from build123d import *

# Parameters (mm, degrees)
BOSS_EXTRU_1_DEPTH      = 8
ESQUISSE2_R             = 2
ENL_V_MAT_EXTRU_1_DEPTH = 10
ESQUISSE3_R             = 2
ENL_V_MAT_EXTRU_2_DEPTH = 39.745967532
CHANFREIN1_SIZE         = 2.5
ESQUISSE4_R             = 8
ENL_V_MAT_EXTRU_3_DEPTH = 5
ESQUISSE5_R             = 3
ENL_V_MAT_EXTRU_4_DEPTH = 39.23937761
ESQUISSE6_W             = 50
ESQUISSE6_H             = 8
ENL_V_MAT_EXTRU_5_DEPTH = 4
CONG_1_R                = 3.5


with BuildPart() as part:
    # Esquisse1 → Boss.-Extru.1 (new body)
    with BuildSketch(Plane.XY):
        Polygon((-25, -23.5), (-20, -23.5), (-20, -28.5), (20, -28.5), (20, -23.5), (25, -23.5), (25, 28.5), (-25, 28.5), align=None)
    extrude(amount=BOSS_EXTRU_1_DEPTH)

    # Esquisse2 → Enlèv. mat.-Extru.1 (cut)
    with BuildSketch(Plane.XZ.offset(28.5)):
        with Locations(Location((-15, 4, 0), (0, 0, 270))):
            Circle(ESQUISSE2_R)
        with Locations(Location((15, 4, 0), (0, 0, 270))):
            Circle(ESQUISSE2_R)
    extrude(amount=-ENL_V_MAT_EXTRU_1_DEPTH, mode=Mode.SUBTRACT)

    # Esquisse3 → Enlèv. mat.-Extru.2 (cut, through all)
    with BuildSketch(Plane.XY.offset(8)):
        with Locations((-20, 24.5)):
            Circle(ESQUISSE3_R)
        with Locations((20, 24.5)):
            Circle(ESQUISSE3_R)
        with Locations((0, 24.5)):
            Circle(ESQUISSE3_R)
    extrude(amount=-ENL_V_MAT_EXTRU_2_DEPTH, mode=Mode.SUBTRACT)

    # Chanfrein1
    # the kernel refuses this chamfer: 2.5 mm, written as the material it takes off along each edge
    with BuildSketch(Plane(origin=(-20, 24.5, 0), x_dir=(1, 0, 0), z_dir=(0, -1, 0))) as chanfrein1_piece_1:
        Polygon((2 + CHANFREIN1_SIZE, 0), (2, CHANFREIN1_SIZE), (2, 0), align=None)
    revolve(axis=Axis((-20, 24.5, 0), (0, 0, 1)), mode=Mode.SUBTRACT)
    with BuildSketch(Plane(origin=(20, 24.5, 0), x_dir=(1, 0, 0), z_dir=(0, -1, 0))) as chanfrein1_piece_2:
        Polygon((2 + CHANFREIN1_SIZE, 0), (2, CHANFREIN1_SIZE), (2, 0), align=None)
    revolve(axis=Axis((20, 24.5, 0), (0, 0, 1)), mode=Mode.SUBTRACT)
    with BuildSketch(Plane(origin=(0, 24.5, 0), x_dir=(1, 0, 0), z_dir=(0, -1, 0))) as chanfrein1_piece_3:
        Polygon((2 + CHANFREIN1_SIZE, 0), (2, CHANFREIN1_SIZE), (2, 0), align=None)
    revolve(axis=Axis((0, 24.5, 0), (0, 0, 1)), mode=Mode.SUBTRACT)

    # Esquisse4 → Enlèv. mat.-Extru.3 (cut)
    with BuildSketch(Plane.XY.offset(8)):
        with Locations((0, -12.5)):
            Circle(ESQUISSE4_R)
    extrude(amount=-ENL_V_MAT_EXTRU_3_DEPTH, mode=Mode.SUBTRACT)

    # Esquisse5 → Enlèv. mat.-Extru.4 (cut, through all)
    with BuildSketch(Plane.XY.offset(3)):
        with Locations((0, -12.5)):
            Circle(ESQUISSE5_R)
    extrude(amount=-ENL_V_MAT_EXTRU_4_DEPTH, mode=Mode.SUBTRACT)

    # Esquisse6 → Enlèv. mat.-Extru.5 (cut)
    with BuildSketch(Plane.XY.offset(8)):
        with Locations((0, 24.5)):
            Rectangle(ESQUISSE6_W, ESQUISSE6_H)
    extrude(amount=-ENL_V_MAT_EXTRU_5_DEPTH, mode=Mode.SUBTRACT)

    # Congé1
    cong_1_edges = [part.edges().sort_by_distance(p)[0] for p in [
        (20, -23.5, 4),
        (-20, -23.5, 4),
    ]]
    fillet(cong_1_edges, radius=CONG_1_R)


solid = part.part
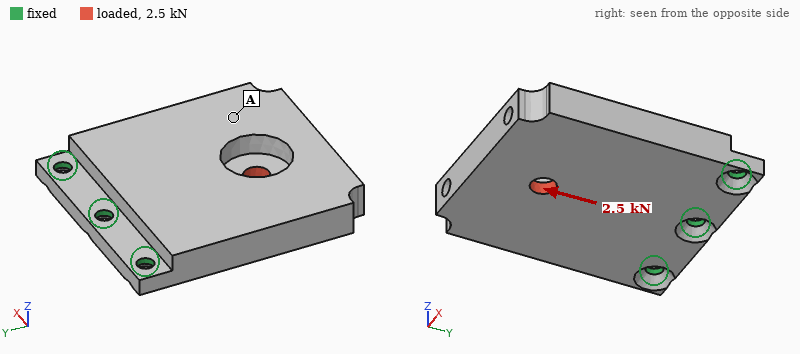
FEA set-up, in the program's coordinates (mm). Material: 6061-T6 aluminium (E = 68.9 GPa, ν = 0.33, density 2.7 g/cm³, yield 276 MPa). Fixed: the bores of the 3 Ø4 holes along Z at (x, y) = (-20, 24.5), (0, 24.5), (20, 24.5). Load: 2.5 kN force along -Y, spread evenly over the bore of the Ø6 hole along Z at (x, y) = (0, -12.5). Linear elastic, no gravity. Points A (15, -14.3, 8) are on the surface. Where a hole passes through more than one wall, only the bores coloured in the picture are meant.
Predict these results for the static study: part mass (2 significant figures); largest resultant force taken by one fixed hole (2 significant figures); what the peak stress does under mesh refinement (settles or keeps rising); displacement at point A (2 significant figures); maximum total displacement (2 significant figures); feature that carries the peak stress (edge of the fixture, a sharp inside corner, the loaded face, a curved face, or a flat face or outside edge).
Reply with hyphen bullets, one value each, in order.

- 52 g
- 910 N
- keeps rising
- 0.11 mm
- 0.17 mm
- edge of the fixture
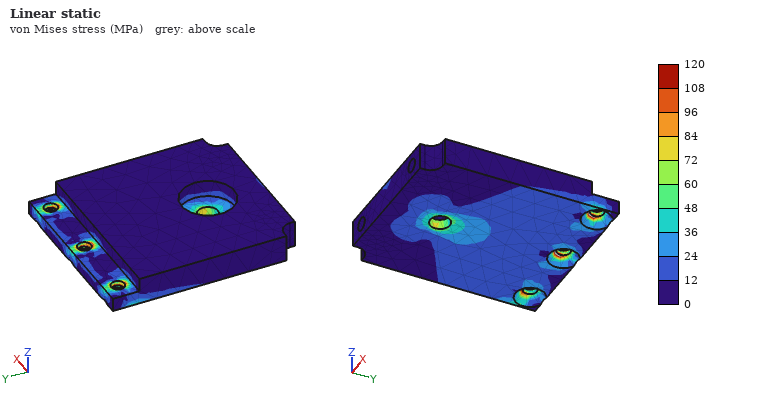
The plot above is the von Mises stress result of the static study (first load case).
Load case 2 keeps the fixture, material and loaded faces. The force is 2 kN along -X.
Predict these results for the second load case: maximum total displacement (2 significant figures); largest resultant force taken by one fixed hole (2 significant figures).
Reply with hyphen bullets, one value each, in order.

- 46 µm
- 1.9 kN
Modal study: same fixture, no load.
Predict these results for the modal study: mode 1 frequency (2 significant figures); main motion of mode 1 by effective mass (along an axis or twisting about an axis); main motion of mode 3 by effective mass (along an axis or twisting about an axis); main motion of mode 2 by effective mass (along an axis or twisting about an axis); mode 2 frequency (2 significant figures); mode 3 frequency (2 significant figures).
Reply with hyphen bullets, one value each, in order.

- 890 Hz
- along Z
- along X
- twisting about Y
- 4400 Hz
- 7600 Hz
